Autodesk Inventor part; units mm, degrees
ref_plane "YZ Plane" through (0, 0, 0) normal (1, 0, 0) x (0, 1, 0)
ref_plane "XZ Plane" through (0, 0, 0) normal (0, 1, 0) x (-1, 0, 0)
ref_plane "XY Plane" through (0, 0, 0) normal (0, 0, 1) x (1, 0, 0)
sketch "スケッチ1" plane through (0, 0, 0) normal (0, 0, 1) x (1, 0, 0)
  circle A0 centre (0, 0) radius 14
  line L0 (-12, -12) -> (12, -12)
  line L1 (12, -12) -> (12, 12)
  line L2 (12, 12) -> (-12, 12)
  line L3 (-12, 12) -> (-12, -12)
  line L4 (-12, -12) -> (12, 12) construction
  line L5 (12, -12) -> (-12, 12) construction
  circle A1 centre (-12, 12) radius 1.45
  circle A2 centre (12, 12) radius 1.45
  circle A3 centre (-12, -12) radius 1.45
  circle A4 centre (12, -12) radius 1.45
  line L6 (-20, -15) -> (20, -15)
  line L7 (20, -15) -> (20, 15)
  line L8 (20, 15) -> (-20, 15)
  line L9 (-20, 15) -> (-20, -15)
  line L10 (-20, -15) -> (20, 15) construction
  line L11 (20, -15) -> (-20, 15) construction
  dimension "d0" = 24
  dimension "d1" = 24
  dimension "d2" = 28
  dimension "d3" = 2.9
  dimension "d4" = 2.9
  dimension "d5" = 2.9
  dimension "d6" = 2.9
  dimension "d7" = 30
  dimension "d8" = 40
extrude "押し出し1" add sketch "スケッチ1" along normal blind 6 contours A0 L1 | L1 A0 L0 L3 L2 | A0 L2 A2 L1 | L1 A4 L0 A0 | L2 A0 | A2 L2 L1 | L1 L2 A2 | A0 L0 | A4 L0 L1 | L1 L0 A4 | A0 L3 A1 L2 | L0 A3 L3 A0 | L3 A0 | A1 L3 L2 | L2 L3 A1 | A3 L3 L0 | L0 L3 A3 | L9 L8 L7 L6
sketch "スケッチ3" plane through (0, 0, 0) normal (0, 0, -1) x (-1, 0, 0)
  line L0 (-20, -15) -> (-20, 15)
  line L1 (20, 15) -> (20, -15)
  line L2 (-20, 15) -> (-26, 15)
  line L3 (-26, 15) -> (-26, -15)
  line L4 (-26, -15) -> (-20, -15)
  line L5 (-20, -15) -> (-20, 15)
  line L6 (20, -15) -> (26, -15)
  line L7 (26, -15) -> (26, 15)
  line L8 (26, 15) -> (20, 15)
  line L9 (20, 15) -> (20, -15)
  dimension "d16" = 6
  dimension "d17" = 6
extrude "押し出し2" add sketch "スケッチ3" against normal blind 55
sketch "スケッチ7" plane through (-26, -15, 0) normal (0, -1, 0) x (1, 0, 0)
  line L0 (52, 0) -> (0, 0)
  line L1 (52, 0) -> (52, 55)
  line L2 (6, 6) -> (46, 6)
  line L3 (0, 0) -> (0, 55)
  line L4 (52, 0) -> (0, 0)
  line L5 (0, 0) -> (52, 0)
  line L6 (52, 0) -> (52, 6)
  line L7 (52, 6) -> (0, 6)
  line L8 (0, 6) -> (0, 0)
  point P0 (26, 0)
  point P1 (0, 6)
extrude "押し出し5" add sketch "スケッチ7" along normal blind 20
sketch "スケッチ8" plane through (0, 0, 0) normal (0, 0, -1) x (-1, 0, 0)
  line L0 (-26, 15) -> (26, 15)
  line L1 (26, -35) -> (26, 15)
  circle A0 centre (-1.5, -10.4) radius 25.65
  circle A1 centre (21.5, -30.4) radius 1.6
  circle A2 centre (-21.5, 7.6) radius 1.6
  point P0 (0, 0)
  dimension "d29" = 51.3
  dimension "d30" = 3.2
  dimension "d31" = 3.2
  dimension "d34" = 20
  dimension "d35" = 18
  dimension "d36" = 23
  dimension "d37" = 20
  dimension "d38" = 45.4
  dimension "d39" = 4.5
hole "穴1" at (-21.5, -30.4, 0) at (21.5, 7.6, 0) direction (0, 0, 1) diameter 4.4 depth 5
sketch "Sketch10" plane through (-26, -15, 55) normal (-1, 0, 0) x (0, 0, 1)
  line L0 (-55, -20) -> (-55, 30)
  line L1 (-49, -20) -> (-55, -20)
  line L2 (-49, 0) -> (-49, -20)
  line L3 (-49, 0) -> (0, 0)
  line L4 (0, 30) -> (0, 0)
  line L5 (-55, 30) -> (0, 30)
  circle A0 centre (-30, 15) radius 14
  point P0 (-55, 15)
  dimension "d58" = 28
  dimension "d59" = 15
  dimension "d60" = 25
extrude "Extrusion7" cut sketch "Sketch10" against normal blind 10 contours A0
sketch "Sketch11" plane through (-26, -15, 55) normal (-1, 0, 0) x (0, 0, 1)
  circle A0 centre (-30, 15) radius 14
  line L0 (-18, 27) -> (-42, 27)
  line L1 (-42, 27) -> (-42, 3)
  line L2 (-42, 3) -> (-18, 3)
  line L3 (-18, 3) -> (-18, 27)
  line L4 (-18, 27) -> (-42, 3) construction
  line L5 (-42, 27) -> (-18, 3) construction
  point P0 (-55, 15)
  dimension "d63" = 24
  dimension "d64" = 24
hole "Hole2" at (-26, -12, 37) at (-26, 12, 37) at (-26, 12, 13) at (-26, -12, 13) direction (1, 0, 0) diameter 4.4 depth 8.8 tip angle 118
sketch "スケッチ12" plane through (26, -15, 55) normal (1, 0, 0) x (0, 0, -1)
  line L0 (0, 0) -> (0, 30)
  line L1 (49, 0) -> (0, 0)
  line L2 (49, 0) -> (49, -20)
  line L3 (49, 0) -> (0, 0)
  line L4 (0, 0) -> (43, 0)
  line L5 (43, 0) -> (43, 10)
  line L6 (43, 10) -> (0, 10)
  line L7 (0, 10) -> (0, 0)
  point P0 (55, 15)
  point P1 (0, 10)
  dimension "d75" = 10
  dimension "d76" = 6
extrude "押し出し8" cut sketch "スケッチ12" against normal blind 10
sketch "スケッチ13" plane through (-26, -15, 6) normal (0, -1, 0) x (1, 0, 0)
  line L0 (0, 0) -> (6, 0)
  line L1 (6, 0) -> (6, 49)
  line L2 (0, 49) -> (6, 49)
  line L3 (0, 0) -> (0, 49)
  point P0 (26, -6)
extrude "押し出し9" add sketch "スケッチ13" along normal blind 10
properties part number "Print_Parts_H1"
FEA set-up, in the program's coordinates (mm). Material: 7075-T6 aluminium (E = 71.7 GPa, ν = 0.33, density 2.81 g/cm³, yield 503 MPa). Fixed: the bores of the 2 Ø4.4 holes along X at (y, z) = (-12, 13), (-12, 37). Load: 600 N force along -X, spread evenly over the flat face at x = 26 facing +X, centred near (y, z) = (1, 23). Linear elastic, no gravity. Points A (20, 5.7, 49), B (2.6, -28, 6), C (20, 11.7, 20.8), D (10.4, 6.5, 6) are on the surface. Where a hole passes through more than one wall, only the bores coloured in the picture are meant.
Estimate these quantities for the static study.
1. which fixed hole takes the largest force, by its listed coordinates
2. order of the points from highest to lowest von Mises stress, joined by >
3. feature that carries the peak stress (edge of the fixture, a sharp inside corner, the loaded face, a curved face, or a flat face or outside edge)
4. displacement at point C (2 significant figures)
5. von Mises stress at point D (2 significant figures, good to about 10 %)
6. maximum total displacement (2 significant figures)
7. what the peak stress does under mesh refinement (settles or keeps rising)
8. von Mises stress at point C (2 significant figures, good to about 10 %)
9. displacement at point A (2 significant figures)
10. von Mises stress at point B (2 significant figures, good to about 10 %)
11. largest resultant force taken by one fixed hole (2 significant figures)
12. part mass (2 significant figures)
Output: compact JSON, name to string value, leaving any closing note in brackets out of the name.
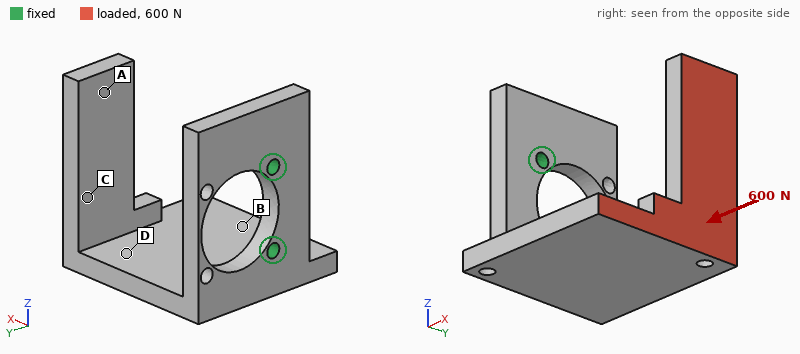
{"which fixed hole takes the largest force, by its listed coordinates": "(-12, 13)", "order of the points from highest to lowest von Mises stress, joined by >": "D > C > B > A", "feature that carries the peak stress": "edge of the fixture", "displacement at point C": "0.41 mm", "von Mises stress at point D": "54 MPa", "maximum total displacement": "1.0 mm", "what the peak stress does under mesh refinement": "keeps rising", "von Mises stress at point C": "42 MPa", "displacement at point A": "0.85 mm", "von Mises stress at point B": "32 MPa", "largest resultant force taken by one fixed hole": "500 N", "part mass": "83 g"}
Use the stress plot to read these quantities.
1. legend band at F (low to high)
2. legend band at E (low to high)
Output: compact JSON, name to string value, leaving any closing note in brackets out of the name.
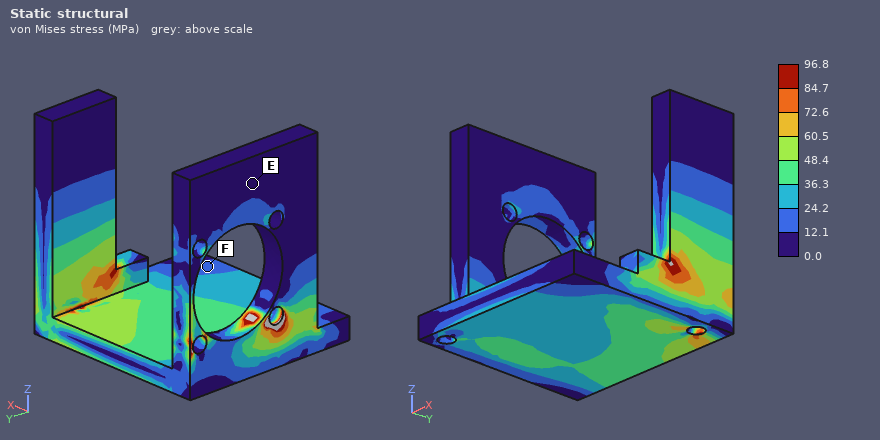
{"legend band at F": "12.1 to 24.2 MPa", "legend band at E": "0.0 to 12.1 MPa"}
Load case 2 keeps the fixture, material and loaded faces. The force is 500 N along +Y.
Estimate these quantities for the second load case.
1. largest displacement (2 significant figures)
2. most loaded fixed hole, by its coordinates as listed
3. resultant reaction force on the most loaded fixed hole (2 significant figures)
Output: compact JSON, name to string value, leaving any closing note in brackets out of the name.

{"largest displacement": "0.69 mm", "most loaded fixed hole, by its coordinates as listed": "(-12, 13)", "resultant reaction force on the most loaded fixed hole": "400 N"}
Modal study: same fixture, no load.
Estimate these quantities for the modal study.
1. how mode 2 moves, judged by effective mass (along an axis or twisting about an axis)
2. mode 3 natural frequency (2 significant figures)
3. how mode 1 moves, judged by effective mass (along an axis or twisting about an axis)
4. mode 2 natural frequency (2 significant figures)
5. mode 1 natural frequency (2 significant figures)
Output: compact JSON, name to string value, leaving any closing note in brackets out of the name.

{"how mode 2 moves, judged by effective mass": "along Y", "mode 3 natural frequency": "1700 Hz", "how mode 1 moves, judged by effective mass": "along Z", "mode 2 natural frequency": "980 Hz", "mode 1 natural frequency": "700 Hz"}
